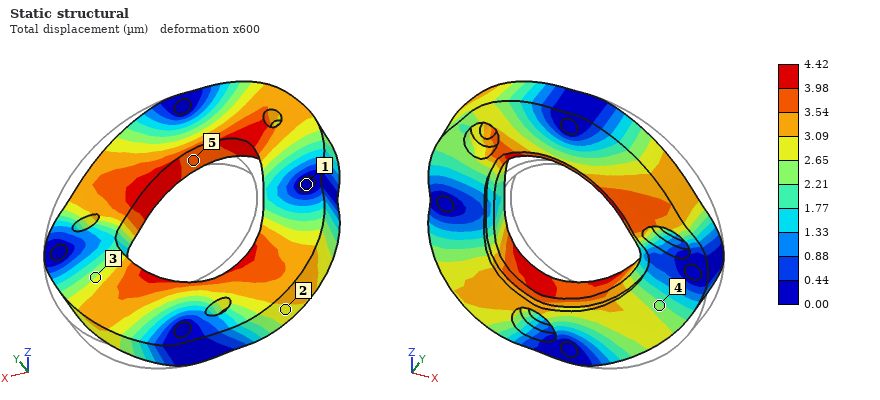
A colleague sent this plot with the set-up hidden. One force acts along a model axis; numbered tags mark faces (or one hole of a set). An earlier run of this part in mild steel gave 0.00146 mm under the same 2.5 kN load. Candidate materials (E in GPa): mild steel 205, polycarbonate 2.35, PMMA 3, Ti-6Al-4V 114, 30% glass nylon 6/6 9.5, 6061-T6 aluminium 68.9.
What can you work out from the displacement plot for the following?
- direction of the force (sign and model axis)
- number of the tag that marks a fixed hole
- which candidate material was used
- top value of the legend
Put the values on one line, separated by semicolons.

-X; 1; 6061-T6 aluminium; 4.42 µm
